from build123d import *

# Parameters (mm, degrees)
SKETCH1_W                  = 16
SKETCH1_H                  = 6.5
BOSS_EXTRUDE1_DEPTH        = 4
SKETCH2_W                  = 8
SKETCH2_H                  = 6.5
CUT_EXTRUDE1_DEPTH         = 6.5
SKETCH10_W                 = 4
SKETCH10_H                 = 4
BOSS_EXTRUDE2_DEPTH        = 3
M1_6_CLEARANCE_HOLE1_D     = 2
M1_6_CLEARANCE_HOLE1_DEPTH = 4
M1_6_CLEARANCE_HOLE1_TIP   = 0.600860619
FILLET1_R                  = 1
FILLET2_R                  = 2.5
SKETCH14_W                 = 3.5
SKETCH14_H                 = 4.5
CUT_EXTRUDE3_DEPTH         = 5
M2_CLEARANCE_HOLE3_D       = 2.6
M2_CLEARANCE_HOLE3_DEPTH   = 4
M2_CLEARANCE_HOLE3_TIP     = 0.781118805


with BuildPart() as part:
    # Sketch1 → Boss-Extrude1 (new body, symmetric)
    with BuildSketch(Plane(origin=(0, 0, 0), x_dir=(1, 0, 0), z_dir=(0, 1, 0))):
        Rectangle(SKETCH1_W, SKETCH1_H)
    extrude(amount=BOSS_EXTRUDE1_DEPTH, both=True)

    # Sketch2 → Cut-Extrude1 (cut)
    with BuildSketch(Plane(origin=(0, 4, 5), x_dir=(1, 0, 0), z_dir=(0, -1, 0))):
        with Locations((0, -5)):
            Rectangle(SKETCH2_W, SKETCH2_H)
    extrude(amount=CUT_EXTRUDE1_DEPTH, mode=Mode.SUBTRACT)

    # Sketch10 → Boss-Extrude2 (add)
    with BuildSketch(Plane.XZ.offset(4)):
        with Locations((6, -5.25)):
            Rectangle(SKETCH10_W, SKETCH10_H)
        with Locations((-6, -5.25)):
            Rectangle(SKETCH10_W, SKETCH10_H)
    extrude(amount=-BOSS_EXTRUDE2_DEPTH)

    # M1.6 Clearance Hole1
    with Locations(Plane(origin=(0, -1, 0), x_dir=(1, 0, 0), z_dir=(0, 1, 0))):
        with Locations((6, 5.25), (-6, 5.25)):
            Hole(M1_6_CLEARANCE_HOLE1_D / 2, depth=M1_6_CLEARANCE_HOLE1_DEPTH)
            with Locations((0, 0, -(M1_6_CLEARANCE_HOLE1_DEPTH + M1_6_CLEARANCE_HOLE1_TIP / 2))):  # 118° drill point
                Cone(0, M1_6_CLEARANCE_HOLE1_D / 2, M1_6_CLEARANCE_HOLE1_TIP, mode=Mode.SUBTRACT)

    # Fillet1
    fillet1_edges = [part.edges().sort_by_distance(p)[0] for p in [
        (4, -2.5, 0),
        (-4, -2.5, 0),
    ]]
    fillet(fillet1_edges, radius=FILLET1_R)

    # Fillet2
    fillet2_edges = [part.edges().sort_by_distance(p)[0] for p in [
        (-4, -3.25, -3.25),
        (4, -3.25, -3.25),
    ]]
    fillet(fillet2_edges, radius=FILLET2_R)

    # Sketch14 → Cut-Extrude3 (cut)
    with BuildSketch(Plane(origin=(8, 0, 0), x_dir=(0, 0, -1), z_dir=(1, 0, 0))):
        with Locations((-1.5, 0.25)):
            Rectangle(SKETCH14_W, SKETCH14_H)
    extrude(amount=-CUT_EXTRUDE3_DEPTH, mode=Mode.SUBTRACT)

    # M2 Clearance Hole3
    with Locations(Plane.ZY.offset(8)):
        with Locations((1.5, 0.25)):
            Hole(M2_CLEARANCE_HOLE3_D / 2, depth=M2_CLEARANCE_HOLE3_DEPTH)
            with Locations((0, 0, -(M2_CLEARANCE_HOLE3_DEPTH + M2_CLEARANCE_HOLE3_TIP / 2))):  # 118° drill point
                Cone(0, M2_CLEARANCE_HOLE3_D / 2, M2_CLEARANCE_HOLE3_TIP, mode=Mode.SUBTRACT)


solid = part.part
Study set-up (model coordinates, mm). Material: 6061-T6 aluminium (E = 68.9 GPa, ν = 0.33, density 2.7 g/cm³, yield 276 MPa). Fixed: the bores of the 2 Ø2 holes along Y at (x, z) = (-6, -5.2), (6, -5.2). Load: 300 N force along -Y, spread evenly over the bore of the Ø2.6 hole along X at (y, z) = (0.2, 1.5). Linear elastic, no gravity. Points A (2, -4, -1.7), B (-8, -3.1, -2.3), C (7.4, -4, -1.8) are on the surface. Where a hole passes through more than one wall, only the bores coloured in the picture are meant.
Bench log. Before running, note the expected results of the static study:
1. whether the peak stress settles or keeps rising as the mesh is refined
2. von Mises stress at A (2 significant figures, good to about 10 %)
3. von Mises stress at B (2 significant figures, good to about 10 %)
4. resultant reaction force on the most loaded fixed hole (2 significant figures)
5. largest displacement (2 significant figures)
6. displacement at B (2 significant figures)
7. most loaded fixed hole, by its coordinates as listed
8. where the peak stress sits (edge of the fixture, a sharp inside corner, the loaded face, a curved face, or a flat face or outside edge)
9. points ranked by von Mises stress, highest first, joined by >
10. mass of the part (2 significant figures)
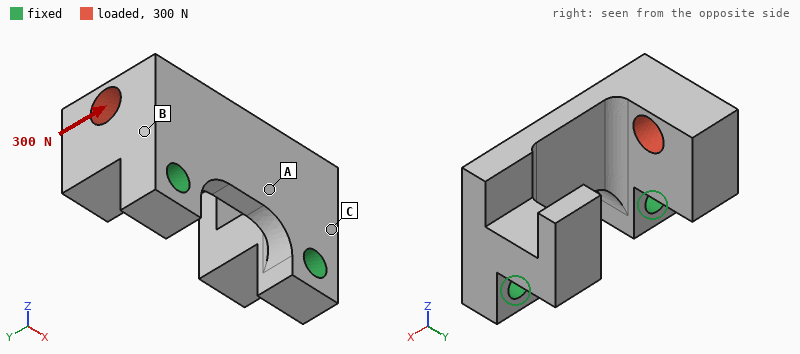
keeps rising
52 MPa
99 MPa
280 N
61 µm
9.7 µm
(-6, -5.2)
edge of the fixture
B > A > C
1.3 g
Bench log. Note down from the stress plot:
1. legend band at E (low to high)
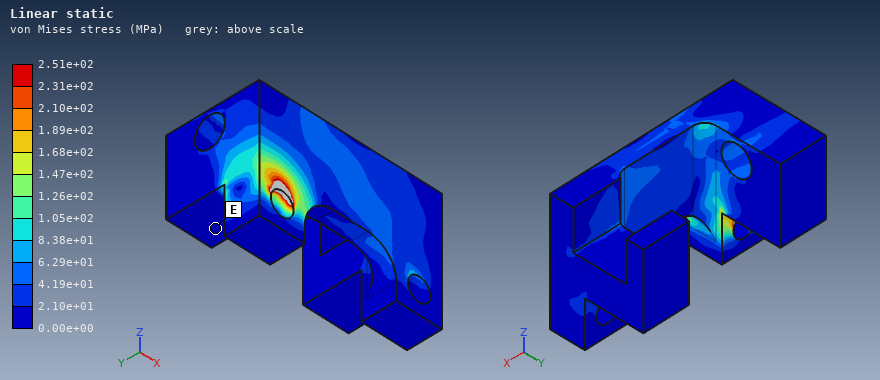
0.00e+00 to 2.10e+01 MPa
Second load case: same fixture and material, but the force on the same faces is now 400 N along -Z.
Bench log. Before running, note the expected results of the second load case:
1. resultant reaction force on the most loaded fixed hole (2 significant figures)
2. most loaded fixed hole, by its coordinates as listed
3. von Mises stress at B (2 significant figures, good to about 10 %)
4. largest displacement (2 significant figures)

410 N
(-6, -5.2)
54 MPa
43 µm
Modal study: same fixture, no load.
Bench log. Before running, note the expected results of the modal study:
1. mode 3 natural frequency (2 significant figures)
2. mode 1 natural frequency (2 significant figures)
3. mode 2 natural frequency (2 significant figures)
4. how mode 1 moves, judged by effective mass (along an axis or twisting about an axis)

26 kHz
19 kHz
23 kHz
along Y
